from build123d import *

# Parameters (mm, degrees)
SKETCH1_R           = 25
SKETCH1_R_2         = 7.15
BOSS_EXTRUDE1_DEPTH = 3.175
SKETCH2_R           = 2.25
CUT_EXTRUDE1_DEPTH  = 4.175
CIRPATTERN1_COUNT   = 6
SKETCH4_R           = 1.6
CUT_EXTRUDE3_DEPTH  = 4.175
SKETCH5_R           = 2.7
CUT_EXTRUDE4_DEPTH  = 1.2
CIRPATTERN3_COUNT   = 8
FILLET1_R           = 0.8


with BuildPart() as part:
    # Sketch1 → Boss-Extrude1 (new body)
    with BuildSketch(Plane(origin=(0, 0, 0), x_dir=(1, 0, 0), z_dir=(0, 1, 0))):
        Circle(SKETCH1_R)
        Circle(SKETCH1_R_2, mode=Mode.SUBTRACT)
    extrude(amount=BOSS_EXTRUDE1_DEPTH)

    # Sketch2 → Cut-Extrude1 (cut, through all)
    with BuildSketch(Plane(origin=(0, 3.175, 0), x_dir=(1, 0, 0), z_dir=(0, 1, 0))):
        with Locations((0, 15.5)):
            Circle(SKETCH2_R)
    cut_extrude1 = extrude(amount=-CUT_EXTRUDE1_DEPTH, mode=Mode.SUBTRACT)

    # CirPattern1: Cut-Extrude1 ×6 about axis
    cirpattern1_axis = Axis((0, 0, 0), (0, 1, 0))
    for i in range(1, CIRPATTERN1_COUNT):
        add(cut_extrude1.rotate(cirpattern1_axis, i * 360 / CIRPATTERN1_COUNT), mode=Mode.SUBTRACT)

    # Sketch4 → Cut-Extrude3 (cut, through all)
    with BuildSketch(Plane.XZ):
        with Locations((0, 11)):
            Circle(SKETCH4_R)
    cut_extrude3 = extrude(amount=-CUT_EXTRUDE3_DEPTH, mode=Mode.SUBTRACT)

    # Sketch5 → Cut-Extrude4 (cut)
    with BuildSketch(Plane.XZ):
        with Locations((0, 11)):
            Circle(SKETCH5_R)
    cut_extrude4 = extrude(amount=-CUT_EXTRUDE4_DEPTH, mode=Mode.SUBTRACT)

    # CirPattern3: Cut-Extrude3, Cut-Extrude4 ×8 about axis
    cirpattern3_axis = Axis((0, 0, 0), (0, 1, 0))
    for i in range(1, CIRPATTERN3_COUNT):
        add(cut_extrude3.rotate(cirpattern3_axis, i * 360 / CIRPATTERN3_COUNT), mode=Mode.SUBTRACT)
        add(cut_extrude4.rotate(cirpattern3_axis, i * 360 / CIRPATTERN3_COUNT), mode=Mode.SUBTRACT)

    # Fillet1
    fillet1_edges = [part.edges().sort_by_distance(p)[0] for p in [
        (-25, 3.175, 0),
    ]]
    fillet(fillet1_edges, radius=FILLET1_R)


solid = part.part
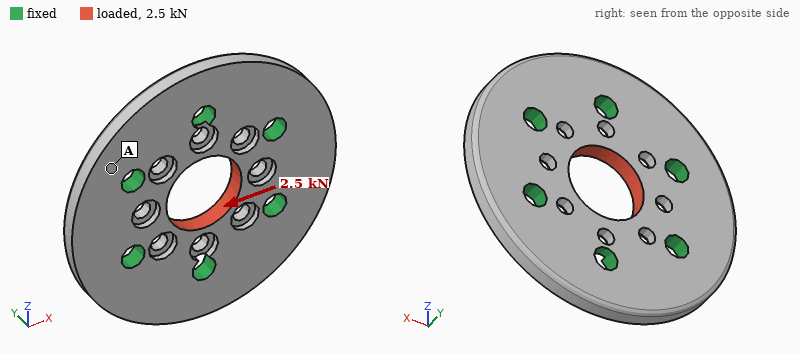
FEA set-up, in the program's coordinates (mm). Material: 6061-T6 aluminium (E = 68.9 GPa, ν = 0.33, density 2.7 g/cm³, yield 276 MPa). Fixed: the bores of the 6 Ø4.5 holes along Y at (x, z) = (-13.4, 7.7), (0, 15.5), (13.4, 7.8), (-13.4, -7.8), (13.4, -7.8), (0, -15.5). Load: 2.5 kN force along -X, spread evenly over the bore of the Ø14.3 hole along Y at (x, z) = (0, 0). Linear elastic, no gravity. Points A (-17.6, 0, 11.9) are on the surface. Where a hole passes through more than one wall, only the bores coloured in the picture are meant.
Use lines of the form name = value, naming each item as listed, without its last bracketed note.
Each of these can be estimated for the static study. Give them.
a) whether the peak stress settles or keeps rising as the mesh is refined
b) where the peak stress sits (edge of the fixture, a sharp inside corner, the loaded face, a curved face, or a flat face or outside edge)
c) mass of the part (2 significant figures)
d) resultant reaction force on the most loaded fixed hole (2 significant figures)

whether the peak stress settles or keeps rising as the mesh is refined = keeps rising
where the peak stress sits = a sharp inside corner
mass of the part = 14 g
resultant reaction force on the most loaded fixed hole = 540 N
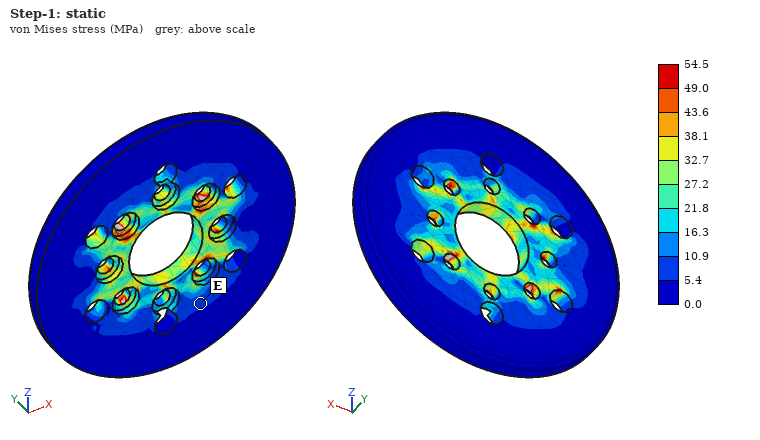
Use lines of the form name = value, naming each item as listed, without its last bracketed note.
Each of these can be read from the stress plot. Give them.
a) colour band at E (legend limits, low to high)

colour band at E = 5.4 to 10.9 MPa
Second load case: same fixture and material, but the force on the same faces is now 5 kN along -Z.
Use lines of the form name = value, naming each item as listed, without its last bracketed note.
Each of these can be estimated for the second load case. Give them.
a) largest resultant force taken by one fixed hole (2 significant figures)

largest resultant force taken by one fixed hole = 1.2 kN
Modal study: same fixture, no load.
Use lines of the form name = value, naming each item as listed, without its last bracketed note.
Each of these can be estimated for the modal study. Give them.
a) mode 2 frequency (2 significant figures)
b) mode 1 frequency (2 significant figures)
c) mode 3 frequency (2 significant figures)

mode 2 frequency = 26 kHz
mode 1 frequency = 25 kHz
mode 3 frequency = 26 kHz
